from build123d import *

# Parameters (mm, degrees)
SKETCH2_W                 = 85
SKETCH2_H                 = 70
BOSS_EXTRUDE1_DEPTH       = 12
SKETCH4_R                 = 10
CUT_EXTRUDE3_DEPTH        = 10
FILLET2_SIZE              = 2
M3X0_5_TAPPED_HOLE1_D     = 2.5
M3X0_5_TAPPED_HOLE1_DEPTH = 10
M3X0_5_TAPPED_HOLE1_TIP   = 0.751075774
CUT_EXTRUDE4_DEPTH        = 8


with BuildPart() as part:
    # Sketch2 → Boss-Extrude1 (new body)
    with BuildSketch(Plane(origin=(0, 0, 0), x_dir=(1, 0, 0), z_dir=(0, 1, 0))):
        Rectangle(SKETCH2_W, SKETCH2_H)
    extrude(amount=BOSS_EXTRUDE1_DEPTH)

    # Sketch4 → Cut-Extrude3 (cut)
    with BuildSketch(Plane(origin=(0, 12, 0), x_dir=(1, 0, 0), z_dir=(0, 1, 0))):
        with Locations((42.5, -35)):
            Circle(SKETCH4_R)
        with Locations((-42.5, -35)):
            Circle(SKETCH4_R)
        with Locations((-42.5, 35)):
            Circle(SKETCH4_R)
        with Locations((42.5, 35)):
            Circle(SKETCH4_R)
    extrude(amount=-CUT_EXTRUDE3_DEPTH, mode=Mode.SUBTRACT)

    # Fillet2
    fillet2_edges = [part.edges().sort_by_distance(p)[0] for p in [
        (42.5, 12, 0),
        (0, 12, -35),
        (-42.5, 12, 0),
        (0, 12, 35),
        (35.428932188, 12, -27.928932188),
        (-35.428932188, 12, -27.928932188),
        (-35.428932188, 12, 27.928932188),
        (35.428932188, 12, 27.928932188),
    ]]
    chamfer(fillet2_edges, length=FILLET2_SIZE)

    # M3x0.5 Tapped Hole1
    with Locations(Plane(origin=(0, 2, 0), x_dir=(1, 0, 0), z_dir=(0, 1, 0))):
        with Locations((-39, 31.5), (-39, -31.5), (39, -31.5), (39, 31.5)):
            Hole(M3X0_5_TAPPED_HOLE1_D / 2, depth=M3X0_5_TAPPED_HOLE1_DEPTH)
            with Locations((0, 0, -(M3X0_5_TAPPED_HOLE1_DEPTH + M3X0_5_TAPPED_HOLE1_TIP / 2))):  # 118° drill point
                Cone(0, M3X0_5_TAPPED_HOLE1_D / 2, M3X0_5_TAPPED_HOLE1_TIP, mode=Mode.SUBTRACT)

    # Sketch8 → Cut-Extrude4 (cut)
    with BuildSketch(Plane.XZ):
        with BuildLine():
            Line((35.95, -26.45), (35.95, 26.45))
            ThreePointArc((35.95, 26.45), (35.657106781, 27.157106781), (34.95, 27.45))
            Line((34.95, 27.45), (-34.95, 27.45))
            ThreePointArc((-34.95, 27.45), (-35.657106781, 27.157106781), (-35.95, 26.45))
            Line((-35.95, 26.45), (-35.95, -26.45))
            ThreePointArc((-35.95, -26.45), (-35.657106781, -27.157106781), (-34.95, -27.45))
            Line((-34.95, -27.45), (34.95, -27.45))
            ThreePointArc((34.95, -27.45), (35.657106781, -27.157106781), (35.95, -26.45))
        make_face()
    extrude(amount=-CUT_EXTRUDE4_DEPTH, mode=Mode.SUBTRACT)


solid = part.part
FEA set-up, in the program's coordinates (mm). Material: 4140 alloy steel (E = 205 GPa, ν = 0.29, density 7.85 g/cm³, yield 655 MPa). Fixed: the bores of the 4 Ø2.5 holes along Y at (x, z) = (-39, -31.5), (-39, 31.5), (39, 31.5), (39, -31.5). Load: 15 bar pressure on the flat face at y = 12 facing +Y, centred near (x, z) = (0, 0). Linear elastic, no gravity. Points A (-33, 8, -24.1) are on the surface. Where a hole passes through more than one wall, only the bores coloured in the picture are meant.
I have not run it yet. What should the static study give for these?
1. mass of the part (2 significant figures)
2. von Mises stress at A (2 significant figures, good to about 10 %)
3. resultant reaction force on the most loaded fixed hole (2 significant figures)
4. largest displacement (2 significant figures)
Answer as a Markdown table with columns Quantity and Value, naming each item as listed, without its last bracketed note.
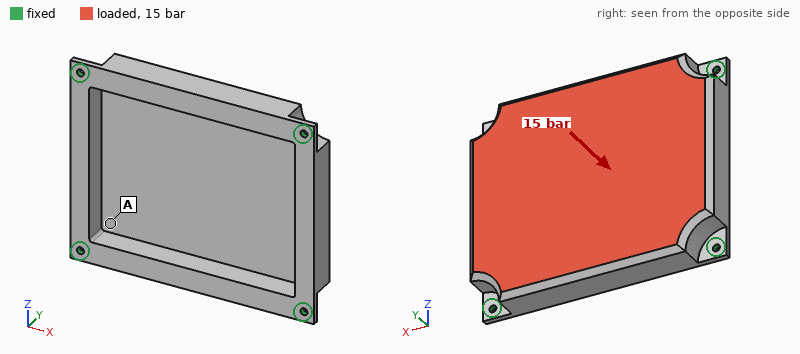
| Quantity | Value |
|---|---|
| mass of the part | 280 g |
| von Mises stress at A | 72 MPa |
| resultant reaction force on the most loaded fixed hole | 3.2 kN |
| largest displacement | 0.10 mm |
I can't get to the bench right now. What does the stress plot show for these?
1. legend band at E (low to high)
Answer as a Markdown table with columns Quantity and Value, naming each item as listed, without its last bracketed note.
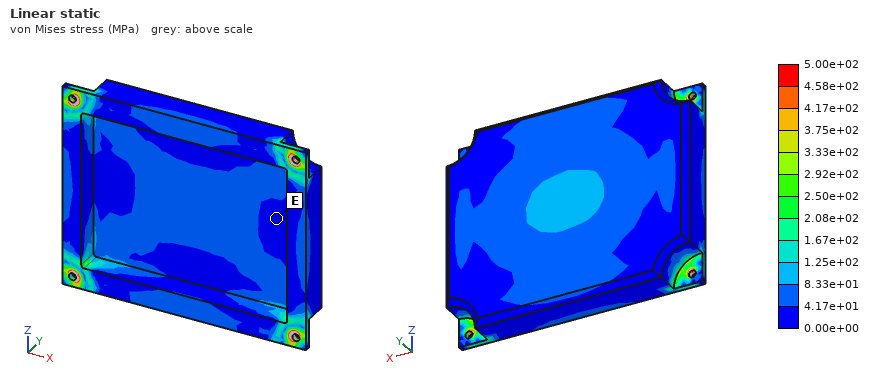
| Quantity | Value |
|---|---|
| legend band at E | 0.00e+00 to 4.17e+01 MPa |
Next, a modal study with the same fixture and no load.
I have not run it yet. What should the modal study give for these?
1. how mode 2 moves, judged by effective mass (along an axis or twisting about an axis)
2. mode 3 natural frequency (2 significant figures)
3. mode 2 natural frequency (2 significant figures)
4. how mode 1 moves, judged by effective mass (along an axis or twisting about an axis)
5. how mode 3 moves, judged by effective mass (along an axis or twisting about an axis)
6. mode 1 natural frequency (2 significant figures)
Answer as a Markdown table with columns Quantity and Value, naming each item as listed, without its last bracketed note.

| Quantity | Value |
|---|---|
| how mode 2 moves, judged by effective mass | twisting about X |
| mode 3 natural frequency | 6100 Hz |
| mode 2 natural frequency | 5100 Hz |
| how mode 1 moves, judged by effective mass | along Y |
| how mode 3 moves, judged by effective mass | twisting about Z |
| mode 1 natural frequency | 3800 Hz |
